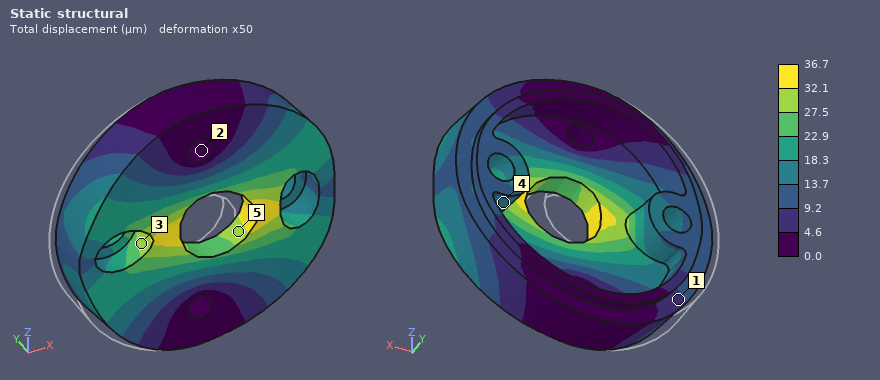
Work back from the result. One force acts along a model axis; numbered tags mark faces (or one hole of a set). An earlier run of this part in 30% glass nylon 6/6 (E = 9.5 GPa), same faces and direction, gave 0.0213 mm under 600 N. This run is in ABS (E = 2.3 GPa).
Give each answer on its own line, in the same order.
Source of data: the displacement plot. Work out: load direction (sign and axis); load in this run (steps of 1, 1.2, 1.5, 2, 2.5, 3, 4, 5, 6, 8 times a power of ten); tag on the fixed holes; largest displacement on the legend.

+X
250 N
2
36.7 µm
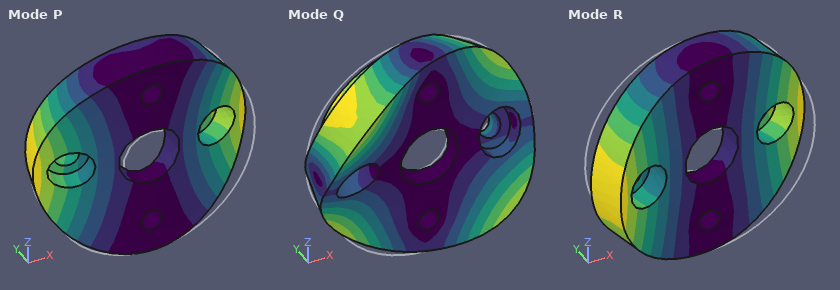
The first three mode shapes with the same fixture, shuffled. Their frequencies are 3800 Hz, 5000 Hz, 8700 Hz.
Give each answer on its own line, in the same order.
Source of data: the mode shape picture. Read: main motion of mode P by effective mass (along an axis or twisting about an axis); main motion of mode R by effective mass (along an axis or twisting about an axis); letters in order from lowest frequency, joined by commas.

along Y
twisting about Z
R, P, Q
